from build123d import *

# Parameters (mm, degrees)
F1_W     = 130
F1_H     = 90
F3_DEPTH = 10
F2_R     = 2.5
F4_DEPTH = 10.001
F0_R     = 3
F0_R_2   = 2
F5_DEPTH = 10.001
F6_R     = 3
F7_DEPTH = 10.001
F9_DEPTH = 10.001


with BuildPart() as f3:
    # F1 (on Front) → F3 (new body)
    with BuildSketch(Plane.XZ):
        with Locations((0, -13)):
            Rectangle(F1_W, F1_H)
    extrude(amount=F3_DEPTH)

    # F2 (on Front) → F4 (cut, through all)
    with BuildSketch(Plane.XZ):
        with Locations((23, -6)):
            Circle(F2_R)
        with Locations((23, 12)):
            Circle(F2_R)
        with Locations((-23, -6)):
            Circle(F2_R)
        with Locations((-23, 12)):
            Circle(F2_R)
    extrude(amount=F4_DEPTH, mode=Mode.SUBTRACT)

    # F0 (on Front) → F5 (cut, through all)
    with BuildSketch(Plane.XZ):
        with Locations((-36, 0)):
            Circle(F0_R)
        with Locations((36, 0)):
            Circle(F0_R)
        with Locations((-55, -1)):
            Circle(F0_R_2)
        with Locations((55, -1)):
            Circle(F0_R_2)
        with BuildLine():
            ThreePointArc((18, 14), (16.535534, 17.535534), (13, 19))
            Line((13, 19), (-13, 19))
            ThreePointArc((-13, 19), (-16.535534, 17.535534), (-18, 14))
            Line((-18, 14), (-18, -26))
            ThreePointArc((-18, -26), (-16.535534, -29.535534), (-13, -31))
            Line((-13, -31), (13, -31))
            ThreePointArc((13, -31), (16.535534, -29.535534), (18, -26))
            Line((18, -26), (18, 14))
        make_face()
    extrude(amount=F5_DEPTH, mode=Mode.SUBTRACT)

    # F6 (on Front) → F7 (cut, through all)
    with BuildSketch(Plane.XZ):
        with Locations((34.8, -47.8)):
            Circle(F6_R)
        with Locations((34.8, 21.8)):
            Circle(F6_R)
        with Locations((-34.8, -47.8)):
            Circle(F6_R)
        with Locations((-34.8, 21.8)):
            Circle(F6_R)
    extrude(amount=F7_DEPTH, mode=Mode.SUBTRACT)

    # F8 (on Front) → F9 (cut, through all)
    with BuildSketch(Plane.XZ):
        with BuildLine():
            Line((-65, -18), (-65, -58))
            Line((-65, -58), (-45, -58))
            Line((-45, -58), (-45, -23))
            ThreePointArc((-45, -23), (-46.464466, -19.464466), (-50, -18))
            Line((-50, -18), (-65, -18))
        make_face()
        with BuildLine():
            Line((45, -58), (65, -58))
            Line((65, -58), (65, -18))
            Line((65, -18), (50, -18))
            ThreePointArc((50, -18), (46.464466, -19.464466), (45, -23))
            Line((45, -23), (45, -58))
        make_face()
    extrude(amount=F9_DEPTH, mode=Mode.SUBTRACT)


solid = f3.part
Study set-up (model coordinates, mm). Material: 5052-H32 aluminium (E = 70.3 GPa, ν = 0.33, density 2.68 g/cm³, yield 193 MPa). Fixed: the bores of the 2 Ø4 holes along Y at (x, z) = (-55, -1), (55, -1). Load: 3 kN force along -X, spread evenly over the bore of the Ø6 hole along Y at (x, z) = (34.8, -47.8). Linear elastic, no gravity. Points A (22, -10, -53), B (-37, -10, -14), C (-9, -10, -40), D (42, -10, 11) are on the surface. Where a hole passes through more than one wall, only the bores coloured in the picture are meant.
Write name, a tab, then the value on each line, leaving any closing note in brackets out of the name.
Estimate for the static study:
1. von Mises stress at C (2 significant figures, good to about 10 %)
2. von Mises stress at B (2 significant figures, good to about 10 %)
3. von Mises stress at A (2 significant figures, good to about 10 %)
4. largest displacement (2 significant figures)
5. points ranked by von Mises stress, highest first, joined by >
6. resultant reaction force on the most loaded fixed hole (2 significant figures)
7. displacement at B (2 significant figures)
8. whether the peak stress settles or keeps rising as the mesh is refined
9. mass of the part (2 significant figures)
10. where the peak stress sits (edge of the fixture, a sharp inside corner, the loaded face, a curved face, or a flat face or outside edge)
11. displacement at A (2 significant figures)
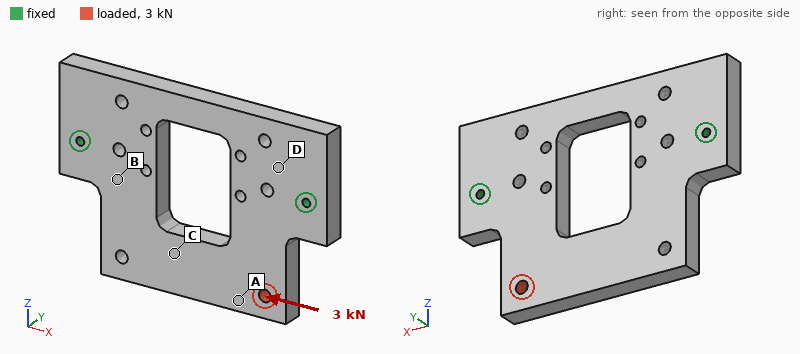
von Mises stress at C	13 MPa
von Mises stress at B	8.4 MPa
von Mises stress at A	16 MPa
largest displacement	22 µm
points ranked by von Mises stress, highest first, joined by >	A > C > B > D
resultant reaction force on the most loaded fixed hole	2.0 kN
displacement at B	4.2 µm
whether the peak stress settles or keeps rising as the mesh is refined	keeps rising
mass of the part	220 g
where the peak stress sits	edge of the fixture
displacement at A	19 µm
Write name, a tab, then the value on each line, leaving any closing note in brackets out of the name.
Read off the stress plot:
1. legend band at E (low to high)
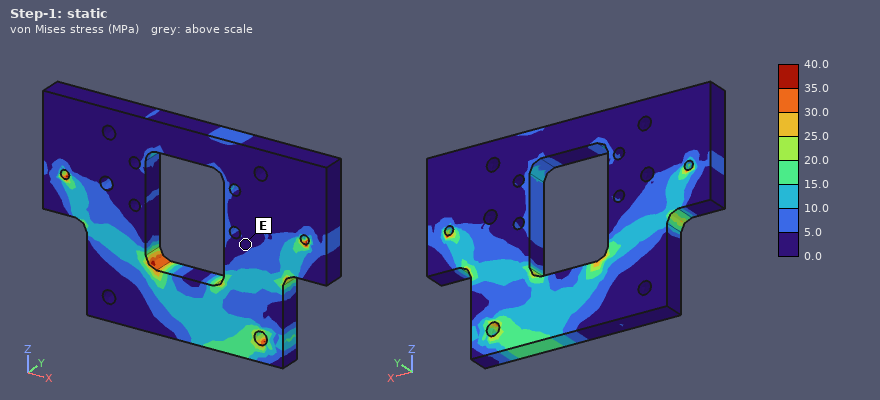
legend band at E	0.0 to 5.0 MPa
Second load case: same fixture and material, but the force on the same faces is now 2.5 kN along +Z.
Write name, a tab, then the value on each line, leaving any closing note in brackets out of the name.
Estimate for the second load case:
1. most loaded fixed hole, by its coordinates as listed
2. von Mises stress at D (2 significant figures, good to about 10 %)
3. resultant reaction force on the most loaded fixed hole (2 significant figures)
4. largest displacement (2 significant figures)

most loaded fixed hole, by its coordinates as listed	(55, -1)
von Mises stress at D	4.1 MPa
resultant reaction force on the most loaded fixed hole	2.1 kN
largest displacement	16 µm
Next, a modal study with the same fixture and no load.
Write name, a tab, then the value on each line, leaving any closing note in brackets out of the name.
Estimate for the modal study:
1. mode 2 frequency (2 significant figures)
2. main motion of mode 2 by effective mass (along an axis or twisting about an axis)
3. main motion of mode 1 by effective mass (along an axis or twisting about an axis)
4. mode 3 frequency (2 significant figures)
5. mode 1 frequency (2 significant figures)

mode 2 frequency	3200 Hz
main motion of mode 2 by effective mass	along Y
main motion of mode 1 by effective mass	along Y
mode 3 frequency	3700 Hz
mode 1 frequency	1500 Hz
